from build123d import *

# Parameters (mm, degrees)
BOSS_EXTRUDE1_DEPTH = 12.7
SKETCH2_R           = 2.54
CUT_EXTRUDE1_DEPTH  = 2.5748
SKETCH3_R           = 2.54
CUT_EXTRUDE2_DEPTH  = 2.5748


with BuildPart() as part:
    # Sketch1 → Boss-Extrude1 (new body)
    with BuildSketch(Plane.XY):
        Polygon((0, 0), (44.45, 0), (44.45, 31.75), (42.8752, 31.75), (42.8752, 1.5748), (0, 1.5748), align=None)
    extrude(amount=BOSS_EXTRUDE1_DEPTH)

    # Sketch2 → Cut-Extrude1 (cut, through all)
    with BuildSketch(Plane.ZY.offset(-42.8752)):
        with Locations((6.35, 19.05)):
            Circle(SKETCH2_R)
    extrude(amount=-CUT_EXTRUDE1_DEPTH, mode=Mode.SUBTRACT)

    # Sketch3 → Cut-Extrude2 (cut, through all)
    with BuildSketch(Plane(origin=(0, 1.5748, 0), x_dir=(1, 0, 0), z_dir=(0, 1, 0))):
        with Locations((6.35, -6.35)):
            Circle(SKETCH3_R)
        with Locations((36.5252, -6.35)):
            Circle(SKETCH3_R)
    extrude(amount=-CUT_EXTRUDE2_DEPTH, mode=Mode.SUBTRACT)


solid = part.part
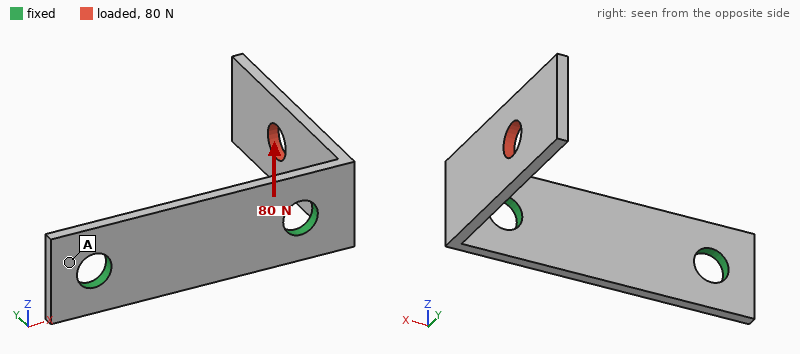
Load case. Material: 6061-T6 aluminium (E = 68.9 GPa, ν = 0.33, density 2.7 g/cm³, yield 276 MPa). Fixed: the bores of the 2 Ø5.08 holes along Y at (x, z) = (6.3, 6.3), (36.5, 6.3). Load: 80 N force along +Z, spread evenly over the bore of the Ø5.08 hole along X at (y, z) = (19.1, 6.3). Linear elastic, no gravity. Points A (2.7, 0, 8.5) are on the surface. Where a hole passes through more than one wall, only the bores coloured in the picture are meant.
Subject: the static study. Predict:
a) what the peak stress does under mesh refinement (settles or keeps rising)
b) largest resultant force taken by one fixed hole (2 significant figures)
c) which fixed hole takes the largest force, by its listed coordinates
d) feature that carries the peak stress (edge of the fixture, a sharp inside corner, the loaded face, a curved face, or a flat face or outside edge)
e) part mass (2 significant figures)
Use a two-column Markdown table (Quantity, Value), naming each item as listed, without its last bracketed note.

| Quantity | Value |
|---|---|
| what the peak stress does under mesh refinement | keeps rising |
| largest resultant force taken by one fixed hole | 85 N |
| which fixed hole takes the largest force, by its listed coordinates | (36.5, 6.3) |
| feature that carries the peak stress | edge of the fixture |
| part mass | 3.8 g |
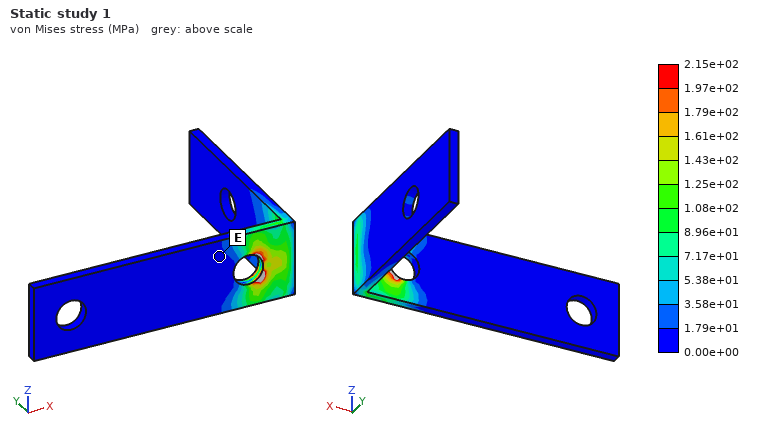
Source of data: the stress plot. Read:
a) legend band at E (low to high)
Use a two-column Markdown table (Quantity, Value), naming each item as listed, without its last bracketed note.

| Quantity | Value |
|---|---|
| legend band at E | 0.00e+00 to 1.79e+01 MPa |
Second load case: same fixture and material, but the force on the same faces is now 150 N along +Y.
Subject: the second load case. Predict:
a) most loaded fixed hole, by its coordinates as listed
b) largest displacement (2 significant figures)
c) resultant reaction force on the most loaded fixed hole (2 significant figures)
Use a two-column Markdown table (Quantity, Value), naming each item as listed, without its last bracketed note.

| Quantity | Value |
|---|---|
| most loaded fixed hole, by its coordinates as listed | (36.5, 6.3) |
| largest displacement | 0.23 mm |
| resultant reaction force on the most loaded fixed hole | 150 N |
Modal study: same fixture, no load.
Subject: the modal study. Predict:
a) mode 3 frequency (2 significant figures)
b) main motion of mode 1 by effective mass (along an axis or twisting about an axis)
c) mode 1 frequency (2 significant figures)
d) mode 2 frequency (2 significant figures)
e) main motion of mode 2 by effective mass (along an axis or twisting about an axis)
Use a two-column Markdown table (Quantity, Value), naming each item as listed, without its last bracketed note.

| Quantity | Value |
|---|---|
| mode 3 frequency | 6200 Hz |
| main motion of mode 1 by effective mass | along X |
| mode 1 frequency | 1100 Hz |
| mode 2 frequency | 2400 Hz |
| main motion of mode 2 by effective mass | along Z |
